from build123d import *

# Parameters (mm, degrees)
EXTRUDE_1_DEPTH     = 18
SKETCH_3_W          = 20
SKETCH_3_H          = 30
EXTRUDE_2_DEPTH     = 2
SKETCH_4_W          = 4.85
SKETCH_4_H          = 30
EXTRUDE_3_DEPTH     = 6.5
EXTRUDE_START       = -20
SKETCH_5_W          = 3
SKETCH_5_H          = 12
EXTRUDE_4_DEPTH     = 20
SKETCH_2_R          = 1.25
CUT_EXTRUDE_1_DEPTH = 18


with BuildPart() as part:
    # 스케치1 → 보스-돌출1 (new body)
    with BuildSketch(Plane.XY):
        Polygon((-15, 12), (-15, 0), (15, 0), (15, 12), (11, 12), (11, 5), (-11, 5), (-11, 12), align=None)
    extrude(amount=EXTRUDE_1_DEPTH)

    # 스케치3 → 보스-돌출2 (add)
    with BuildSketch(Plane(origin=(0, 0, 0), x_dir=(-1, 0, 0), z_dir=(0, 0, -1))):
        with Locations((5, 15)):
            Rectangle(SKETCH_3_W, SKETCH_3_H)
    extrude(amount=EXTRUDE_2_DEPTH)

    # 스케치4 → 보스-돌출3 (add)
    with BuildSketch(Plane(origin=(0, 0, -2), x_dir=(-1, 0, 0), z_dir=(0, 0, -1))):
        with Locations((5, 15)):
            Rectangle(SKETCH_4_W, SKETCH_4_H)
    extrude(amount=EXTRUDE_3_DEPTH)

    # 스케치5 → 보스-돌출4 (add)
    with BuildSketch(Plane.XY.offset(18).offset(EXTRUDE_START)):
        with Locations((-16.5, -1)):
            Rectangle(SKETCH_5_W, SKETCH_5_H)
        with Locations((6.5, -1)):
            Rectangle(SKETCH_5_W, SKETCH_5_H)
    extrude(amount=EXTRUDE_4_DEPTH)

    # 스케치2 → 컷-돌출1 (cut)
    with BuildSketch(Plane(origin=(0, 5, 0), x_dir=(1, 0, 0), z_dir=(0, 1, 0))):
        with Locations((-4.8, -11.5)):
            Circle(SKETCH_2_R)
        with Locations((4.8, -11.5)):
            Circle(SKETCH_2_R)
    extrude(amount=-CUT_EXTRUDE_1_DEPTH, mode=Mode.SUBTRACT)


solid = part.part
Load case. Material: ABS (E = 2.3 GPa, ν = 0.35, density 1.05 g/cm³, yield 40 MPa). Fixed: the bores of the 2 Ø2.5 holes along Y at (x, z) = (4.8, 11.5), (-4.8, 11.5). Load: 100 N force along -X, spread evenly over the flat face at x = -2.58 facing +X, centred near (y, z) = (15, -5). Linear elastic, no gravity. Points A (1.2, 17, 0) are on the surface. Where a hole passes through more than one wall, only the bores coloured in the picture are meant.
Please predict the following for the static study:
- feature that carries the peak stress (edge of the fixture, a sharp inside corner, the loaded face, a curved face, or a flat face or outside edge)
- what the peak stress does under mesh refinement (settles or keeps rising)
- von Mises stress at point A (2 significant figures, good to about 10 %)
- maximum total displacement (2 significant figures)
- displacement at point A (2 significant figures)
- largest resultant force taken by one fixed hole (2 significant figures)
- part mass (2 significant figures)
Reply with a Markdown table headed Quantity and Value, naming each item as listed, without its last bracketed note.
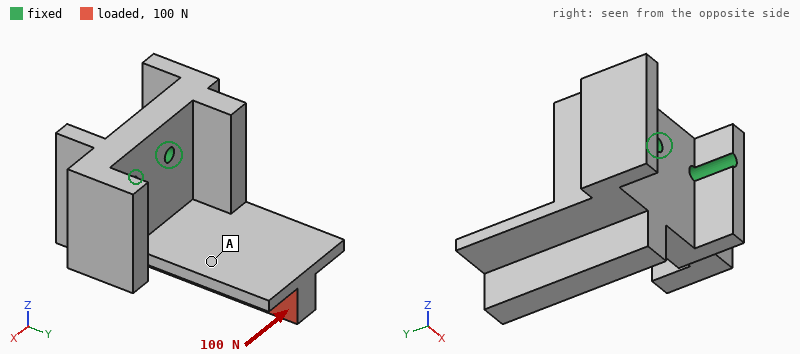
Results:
| Quantity | Value |
|---|---|
| feature that carries the peak stress | edge of the fixture |
| what the peak stress does under mesh refinement | keeps rising |
| von Mises stress at point A | 2.0 MPa |
| maximum total displacement | 0.57 mm |
| displacement at point A | 0.27 mm |
| largest resultant force taken by one fixed hole | 170 N |
| part mass | 7.3 g |
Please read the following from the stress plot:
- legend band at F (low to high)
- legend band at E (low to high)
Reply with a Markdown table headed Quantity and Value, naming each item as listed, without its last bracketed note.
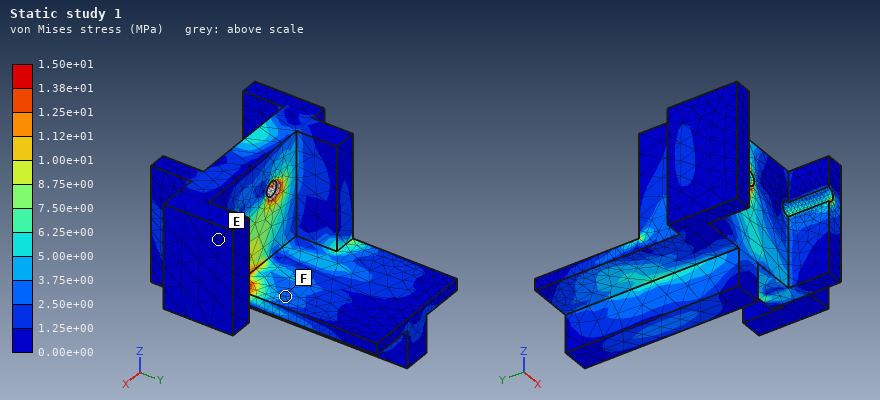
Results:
| Quantity | Value |
|---|---|
| legend band at F | 2.50e+00 to 3.75e+00 MPa |
| legend band at E | 0.00e+00 to 1.25e+00 MPa |
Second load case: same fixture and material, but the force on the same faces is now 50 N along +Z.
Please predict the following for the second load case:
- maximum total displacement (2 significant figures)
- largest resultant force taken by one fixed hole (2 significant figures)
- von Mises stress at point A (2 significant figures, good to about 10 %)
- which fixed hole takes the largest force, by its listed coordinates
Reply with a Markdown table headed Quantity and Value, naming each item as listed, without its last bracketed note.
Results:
| Quantity | Value |
|---|---|
| maximum total displacement | 0.62 mm |
| largest resultant force taken by one fixed hole | 35 N |
| von Mises stress at point A | 2.7 MPa |
| which fixed hole takes the largest force, by its listed coordinates | (-4.8, 11.5) |
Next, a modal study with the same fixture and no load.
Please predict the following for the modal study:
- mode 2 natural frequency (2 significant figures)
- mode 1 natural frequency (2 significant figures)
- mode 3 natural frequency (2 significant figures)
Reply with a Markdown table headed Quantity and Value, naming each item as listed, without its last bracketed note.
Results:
| Quantity | Value |
|---|---|
| mode 2 natural frequency | 1900 Hz |
| mode 1 natural frequency | 1200 Hz |
| mode 3 natural frequency | 3300 Hz |
